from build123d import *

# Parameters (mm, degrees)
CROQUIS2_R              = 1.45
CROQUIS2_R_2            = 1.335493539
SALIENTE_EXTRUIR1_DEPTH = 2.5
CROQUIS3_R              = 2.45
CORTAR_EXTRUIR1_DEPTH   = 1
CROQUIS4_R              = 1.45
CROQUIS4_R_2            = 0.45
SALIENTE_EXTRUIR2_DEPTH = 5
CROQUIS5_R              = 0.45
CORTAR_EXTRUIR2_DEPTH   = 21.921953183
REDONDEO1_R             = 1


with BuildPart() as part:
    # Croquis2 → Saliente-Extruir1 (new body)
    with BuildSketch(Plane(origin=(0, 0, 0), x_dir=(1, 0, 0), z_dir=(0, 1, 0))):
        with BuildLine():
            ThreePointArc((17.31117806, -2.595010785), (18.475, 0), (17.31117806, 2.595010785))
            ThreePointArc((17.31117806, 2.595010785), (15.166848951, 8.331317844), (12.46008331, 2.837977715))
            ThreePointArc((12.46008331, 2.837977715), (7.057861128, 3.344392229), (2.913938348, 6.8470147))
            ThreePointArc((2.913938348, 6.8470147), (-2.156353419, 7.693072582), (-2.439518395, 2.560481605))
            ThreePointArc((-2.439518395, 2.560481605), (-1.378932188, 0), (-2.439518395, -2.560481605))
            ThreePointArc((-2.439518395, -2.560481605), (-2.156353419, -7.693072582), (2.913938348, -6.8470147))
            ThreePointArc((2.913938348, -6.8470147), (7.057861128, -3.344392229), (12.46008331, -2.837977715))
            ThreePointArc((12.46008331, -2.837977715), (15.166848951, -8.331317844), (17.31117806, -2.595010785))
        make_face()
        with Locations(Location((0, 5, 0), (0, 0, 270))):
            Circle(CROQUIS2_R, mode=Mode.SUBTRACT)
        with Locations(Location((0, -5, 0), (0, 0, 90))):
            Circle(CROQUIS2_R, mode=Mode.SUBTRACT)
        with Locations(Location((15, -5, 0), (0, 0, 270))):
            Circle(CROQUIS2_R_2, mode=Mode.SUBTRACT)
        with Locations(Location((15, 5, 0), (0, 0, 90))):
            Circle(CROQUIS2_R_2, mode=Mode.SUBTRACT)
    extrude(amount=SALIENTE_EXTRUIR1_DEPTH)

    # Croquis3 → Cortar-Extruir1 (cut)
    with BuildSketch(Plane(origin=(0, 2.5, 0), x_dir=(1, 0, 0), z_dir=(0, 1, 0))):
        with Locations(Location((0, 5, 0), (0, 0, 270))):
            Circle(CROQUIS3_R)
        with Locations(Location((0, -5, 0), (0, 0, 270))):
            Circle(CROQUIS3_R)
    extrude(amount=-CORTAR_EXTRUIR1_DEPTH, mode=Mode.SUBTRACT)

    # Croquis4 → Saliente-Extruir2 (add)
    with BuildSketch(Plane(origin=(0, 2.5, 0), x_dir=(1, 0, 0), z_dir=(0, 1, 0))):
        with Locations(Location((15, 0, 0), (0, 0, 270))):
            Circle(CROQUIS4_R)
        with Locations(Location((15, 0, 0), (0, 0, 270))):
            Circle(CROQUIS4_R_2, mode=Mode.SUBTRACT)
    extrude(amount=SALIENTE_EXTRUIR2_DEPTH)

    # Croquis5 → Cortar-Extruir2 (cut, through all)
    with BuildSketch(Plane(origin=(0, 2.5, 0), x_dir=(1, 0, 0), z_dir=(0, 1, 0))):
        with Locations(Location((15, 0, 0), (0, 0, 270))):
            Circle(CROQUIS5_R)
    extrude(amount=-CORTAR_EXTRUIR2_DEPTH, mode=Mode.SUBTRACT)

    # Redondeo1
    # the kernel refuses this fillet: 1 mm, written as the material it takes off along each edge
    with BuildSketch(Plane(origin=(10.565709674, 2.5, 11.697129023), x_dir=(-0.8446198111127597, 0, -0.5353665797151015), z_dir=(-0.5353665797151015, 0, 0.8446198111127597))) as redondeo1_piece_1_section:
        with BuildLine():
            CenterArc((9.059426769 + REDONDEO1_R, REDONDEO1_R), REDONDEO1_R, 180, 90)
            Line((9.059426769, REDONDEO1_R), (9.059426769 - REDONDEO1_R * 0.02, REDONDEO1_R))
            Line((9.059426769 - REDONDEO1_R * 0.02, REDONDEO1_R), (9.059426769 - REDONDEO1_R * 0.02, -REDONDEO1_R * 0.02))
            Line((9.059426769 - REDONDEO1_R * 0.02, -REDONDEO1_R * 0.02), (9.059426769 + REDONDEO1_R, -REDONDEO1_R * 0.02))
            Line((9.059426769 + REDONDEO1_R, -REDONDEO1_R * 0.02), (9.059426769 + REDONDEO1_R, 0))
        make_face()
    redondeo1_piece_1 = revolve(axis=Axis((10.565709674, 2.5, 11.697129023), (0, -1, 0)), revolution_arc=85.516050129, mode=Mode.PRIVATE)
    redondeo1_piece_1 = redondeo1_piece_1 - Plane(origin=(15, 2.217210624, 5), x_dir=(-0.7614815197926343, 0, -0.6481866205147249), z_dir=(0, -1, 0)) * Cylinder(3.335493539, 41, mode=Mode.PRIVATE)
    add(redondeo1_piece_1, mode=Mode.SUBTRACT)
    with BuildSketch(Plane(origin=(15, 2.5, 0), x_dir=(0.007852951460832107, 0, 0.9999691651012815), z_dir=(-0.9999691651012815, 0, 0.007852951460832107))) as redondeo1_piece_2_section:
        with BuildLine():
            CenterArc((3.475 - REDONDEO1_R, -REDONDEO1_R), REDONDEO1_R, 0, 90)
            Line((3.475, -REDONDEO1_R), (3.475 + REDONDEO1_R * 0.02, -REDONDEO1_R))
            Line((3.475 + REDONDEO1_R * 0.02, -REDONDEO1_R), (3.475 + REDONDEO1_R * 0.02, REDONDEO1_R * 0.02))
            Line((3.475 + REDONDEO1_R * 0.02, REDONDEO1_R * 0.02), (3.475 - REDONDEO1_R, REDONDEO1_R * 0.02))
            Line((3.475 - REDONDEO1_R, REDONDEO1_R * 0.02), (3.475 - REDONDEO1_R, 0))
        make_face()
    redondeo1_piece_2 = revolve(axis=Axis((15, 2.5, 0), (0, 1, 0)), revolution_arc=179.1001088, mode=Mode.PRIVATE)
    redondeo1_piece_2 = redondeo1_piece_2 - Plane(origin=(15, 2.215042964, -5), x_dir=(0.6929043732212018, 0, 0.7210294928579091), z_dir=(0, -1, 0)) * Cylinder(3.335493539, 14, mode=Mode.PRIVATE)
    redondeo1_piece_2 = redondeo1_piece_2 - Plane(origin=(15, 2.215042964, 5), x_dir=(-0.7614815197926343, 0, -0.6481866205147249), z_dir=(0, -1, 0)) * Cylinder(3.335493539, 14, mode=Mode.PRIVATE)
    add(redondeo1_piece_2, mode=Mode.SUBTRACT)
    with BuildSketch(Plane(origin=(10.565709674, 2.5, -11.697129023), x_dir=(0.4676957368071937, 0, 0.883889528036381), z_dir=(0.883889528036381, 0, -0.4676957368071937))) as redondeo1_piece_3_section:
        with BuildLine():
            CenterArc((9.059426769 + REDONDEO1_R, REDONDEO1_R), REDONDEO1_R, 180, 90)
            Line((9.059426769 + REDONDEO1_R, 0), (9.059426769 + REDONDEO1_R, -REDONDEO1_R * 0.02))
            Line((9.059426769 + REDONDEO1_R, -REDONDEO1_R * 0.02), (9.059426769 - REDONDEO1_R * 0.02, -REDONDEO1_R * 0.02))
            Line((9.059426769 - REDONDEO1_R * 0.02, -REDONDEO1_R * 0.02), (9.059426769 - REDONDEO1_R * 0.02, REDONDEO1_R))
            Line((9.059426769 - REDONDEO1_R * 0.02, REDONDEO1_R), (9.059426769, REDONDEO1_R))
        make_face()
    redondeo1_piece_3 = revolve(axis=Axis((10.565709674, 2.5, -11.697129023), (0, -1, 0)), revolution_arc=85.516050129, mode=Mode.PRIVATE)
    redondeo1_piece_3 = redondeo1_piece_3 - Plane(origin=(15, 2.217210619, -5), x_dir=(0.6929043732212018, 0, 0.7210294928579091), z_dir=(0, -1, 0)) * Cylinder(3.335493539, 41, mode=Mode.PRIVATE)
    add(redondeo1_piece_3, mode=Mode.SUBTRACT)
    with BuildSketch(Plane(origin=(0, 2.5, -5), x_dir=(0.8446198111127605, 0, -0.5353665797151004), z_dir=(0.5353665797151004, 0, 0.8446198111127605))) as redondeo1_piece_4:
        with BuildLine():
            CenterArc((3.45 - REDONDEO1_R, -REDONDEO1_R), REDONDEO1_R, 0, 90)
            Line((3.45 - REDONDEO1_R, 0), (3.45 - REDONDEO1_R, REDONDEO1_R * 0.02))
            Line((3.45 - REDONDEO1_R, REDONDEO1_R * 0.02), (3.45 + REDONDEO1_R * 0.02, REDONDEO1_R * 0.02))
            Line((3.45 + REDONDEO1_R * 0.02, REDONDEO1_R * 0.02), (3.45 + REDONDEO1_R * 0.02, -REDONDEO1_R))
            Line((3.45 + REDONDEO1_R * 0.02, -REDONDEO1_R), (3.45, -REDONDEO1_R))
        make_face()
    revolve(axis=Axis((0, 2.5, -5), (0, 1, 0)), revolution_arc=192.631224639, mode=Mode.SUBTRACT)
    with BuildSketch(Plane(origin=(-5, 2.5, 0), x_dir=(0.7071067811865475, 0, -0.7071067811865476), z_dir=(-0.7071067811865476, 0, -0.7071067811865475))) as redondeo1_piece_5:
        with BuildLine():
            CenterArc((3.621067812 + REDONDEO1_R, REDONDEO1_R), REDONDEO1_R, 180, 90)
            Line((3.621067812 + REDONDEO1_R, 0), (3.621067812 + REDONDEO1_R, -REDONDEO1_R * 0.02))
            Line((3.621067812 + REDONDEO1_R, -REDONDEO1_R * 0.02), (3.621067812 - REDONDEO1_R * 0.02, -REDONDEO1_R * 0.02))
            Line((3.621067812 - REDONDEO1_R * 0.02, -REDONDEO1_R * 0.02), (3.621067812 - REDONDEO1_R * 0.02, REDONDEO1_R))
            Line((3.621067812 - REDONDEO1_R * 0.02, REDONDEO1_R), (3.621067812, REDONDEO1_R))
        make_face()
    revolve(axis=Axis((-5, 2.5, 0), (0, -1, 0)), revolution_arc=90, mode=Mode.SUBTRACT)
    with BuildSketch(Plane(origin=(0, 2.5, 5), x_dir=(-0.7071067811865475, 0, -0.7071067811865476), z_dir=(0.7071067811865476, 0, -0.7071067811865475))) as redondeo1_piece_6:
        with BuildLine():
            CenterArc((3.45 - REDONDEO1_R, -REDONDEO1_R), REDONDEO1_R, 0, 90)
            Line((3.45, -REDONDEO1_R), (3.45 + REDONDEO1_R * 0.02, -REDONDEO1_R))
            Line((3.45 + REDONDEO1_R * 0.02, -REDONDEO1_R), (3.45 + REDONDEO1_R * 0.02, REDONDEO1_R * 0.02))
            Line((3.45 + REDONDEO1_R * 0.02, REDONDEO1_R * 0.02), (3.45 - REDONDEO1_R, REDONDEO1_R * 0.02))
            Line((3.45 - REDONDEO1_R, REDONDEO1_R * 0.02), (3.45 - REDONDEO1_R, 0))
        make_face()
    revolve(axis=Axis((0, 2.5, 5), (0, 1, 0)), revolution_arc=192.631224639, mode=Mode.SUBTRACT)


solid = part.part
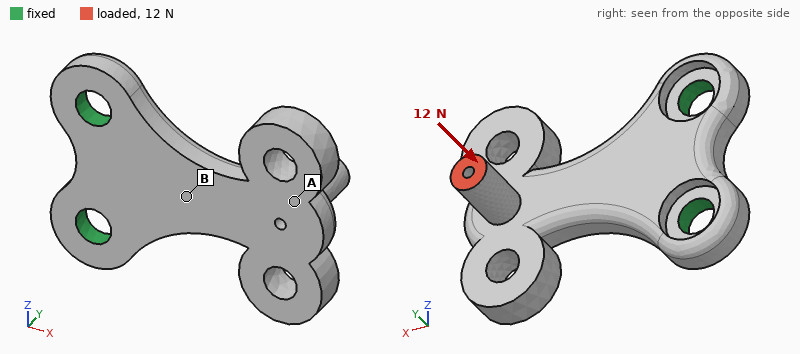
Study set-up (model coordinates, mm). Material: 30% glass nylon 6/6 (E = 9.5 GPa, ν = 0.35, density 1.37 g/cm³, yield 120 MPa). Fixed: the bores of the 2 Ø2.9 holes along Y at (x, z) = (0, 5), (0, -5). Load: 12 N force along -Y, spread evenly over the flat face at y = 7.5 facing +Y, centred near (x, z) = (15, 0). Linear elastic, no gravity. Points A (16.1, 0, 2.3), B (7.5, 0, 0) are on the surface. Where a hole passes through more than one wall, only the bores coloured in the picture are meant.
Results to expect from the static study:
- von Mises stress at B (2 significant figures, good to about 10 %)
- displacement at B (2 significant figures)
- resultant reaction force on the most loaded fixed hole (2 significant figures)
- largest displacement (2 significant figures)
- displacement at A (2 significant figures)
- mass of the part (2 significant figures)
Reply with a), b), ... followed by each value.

a) 15 MPa
b) 0.051 mm
c) 7.0 N
d) 0.22 mm
e) 0.18 mm
f) 0.77 g
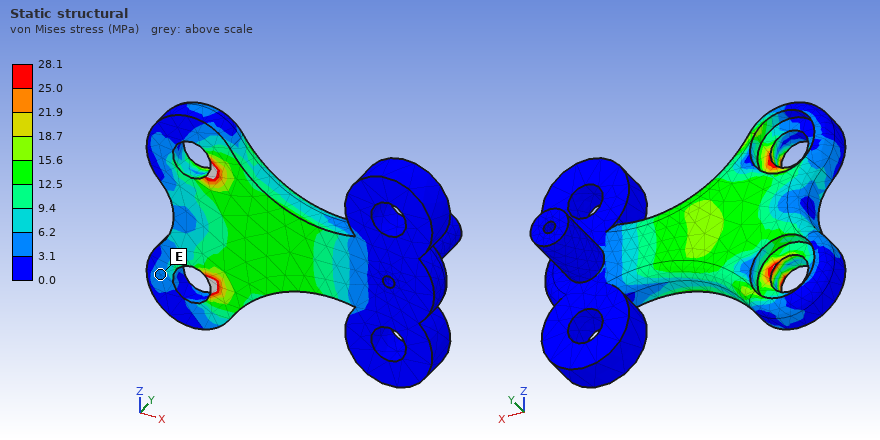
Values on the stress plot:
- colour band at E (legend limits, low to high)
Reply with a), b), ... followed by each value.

a) 3.1 to 6.2 MPa
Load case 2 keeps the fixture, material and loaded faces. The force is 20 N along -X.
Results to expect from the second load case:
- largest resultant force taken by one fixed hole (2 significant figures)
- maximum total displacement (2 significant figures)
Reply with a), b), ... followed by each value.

a) 10 N
b) 0.30 mm
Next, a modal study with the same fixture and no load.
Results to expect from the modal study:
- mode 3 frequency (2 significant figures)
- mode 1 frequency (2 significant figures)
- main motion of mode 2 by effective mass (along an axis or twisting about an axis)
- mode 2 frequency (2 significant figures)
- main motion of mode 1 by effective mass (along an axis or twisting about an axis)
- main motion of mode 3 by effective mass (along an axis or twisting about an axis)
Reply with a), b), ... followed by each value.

a) 6700 Hz
b) 2300 Hz
c) twisting about X
d) 5300 Hz
e) along Y
f) along Z
